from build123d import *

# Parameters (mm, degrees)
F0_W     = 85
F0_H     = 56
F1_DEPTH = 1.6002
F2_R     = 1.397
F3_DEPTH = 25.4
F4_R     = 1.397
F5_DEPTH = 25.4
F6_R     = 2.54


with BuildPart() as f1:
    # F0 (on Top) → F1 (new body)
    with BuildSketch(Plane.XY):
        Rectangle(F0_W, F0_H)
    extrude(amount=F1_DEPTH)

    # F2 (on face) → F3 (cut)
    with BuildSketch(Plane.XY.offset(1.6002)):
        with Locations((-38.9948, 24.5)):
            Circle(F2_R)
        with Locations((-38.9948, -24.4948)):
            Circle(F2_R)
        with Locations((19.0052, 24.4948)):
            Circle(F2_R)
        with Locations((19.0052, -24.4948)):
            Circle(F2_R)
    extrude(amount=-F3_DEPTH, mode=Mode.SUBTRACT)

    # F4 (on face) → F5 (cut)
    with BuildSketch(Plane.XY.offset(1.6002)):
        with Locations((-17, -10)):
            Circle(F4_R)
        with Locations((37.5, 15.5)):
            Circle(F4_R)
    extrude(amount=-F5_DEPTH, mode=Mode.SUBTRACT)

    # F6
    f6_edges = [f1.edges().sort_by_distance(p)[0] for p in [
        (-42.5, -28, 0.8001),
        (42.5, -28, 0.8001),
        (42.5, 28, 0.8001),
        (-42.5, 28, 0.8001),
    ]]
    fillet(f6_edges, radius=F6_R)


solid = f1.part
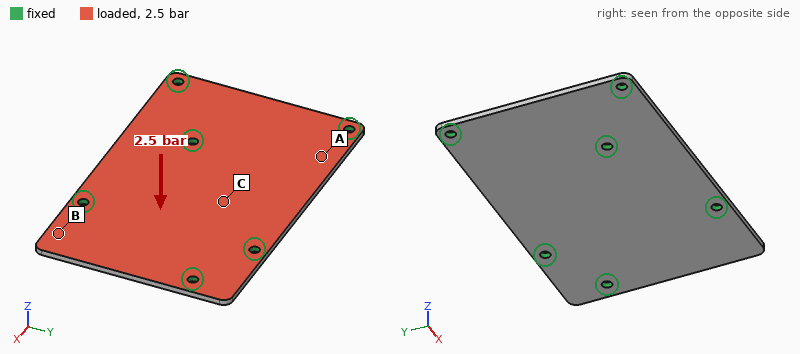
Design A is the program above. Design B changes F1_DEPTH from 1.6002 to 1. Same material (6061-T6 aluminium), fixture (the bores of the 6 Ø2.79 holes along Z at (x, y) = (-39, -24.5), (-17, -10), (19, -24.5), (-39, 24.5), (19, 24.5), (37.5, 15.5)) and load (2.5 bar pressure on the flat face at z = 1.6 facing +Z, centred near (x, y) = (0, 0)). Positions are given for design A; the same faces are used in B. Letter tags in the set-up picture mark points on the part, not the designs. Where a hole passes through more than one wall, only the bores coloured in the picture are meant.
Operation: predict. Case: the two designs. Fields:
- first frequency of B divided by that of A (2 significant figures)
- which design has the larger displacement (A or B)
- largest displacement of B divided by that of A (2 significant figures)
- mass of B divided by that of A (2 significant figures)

0.64
B
4.0
0.62
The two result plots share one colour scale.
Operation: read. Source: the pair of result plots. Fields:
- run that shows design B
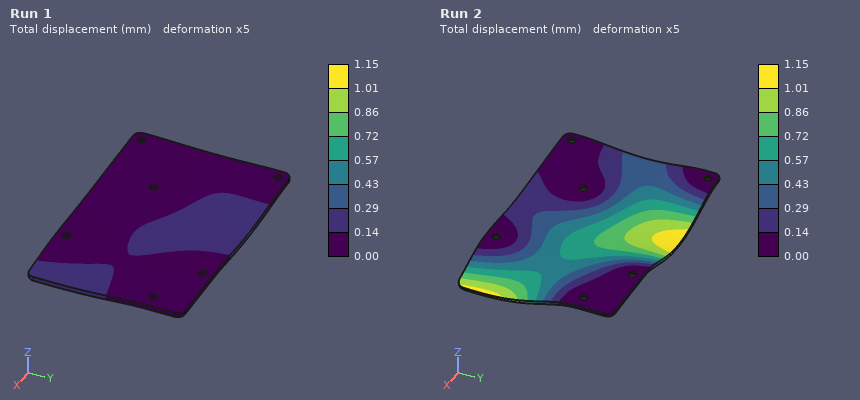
Run 2
